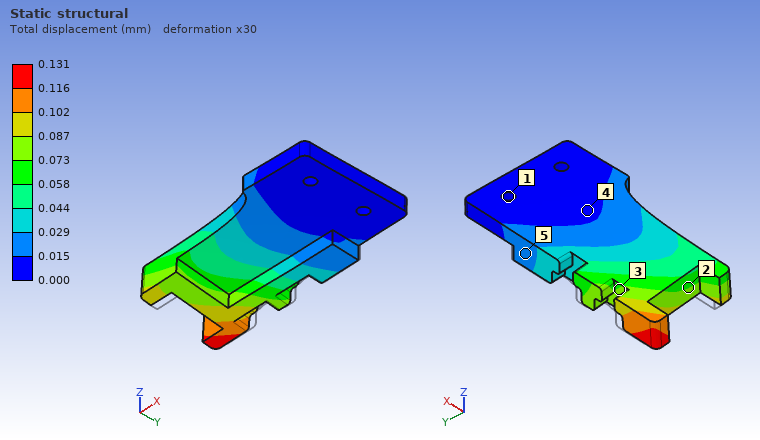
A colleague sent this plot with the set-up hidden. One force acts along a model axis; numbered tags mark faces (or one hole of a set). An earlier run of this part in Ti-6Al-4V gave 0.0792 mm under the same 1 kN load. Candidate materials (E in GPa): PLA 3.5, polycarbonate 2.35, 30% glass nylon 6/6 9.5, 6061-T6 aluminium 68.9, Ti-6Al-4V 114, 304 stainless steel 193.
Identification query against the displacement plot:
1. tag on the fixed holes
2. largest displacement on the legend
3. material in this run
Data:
1
0.131 mm
6061-T6 aluminium
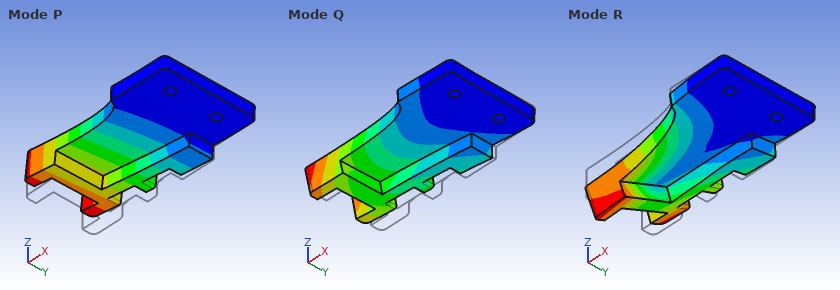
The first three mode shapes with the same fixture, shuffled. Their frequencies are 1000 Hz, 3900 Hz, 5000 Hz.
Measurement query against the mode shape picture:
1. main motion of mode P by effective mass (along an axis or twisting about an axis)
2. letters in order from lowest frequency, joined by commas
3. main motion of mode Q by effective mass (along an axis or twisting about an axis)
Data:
along Z
P, R, Q
along Y
